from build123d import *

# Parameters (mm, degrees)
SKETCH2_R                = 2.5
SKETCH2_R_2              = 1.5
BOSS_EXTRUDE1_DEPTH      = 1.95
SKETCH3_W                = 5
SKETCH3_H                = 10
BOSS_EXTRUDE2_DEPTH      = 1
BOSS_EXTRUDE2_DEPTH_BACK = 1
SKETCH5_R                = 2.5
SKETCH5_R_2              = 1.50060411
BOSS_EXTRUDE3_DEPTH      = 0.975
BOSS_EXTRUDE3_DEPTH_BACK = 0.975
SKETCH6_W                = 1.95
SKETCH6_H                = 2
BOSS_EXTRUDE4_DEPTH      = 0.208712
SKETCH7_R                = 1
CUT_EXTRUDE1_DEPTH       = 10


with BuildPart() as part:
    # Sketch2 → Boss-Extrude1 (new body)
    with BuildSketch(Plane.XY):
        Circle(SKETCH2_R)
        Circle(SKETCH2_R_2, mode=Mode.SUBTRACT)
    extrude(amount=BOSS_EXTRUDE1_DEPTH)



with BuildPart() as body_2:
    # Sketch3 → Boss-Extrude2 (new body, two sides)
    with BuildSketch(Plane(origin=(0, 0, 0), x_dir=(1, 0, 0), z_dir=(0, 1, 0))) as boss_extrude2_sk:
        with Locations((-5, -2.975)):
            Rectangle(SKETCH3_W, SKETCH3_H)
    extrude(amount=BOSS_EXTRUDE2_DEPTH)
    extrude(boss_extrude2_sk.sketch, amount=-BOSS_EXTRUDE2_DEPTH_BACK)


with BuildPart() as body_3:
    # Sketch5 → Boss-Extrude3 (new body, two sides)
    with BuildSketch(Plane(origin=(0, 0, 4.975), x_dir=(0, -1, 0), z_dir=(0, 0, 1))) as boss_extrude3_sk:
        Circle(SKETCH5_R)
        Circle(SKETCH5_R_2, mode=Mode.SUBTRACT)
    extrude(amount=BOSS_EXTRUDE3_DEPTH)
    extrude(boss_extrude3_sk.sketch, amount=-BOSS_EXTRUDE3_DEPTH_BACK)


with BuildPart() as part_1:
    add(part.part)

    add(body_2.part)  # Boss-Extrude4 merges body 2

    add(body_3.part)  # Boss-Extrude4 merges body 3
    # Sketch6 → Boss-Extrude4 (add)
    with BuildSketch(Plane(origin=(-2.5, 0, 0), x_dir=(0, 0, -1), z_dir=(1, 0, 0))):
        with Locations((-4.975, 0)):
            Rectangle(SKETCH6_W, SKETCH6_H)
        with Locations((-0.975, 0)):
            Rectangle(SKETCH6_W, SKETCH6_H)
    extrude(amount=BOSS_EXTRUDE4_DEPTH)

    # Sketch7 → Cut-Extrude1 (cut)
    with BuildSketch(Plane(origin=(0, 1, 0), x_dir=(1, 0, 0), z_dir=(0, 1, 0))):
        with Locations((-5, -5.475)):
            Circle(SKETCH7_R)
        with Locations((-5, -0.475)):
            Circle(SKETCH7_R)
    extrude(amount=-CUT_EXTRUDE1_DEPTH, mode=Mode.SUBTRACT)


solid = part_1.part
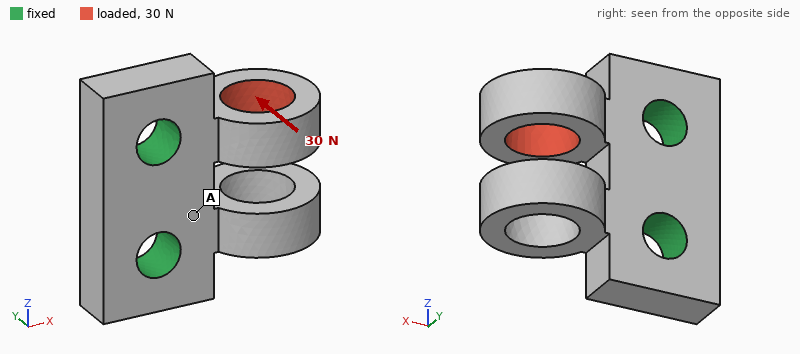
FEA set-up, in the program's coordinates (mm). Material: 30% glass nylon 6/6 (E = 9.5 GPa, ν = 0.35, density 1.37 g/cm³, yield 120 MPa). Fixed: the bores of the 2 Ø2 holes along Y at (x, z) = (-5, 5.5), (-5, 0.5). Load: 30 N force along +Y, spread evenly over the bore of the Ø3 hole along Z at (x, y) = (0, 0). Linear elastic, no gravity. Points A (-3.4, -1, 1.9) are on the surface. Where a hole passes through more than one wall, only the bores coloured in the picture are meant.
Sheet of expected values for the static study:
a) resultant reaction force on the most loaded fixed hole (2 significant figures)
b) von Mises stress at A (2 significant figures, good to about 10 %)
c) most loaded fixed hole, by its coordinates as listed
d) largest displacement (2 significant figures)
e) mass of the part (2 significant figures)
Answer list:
30 N
9.0 MPa
(-5, 5.5)
0.13 mm
0.19 g
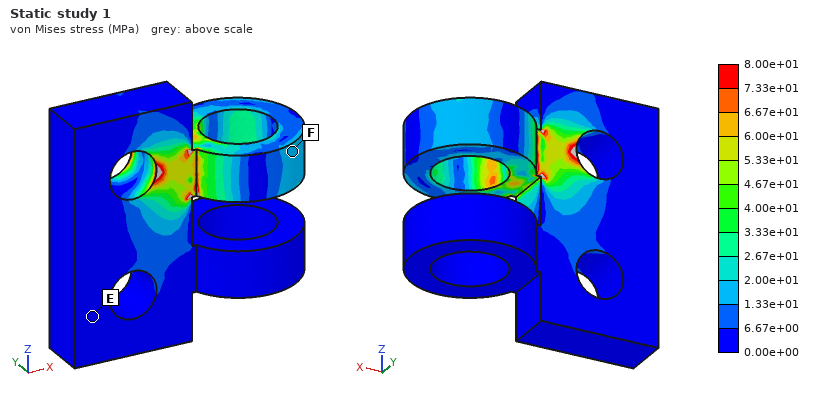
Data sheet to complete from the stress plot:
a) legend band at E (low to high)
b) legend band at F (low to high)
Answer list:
0.00e+00 to 6.67e+00 MPa
1.33e+01 to 2.00e+01 MPa
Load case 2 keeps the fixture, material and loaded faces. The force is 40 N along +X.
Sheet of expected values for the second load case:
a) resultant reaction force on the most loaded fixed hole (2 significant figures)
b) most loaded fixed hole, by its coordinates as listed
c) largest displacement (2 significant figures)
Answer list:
36 N
(-5, 5.5)
15 µm
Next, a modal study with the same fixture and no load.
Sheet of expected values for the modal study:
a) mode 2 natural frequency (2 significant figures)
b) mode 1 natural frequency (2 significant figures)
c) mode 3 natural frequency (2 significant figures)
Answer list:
15 kHz
14 kHz
18 kHz
